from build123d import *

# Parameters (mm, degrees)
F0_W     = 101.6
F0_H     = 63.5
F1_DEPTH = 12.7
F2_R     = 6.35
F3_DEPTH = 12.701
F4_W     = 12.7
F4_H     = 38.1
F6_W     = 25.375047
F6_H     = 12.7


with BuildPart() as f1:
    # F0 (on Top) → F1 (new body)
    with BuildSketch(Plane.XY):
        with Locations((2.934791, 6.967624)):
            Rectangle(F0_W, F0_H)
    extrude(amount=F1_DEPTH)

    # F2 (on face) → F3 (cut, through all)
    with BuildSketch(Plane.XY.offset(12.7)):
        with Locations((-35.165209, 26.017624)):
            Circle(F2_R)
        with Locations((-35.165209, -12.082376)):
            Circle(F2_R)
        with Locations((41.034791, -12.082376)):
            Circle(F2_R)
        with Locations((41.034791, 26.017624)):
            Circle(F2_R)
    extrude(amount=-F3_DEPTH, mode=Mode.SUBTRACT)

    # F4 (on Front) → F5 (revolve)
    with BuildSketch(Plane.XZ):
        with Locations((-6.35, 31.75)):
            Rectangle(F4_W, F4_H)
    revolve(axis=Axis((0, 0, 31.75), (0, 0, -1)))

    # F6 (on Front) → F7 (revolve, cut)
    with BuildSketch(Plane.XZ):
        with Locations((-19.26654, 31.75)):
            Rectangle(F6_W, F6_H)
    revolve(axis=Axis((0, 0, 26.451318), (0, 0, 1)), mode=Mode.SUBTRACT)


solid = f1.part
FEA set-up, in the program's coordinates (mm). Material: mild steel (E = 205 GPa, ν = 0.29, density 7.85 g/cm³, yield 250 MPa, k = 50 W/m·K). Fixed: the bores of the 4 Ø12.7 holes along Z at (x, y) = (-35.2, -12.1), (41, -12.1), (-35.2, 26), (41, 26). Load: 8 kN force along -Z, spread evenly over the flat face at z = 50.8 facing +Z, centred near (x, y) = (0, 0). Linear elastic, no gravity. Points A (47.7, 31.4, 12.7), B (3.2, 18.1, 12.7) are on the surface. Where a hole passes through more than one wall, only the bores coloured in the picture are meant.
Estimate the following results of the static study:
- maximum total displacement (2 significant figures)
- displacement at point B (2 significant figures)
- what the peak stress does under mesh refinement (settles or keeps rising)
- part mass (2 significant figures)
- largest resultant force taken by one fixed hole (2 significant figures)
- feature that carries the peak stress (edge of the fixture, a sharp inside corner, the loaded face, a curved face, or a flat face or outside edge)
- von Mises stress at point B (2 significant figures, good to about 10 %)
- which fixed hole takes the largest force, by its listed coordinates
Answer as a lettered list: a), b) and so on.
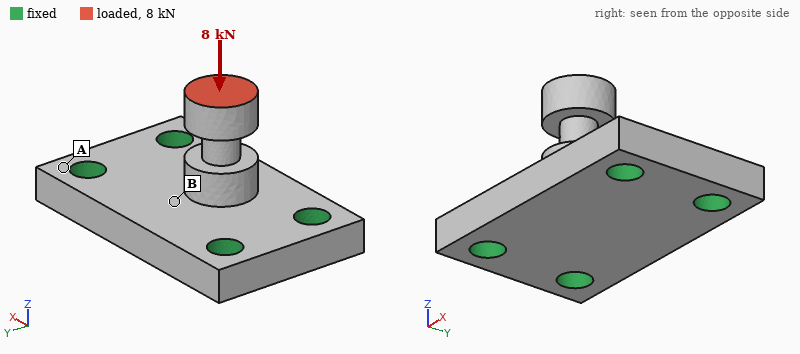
a) 16 µm
b) 5.9 µm
c) keeps rising
d) 710 g
e) 3.0 kN
f) edge of the fixture
g) 17 MPa
h) (-35.2, -12.1)
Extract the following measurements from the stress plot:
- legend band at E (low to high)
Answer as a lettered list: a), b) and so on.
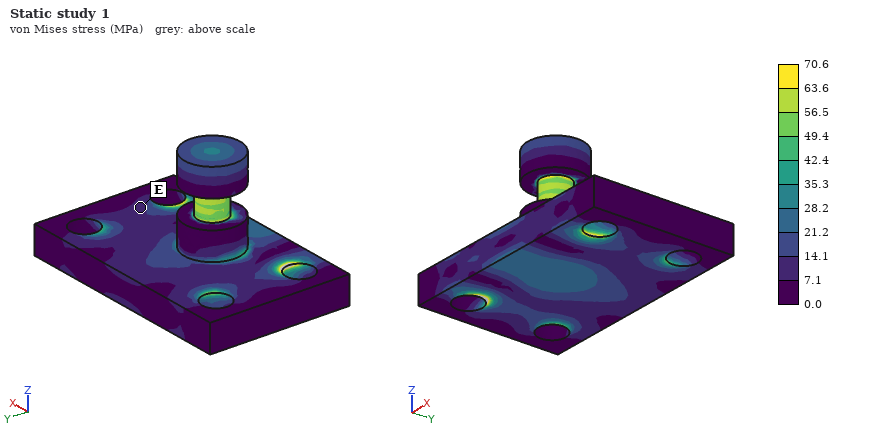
a) 7.1 to 14.1 MPa
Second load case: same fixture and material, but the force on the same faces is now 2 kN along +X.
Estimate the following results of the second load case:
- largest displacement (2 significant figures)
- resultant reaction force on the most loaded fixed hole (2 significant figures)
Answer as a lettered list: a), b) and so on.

a) 73 µm
b) 1.4 kN
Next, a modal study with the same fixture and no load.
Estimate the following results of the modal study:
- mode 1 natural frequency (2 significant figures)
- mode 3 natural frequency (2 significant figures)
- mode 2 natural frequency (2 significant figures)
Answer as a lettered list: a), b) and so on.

a) 4600 Hz
b) 9100 Hz
c) 4800 Hz
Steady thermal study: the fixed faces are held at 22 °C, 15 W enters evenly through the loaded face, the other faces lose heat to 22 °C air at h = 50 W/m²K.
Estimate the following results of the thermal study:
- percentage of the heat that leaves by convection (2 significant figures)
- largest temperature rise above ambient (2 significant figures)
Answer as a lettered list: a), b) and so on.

a) 35 %
b) 46 K
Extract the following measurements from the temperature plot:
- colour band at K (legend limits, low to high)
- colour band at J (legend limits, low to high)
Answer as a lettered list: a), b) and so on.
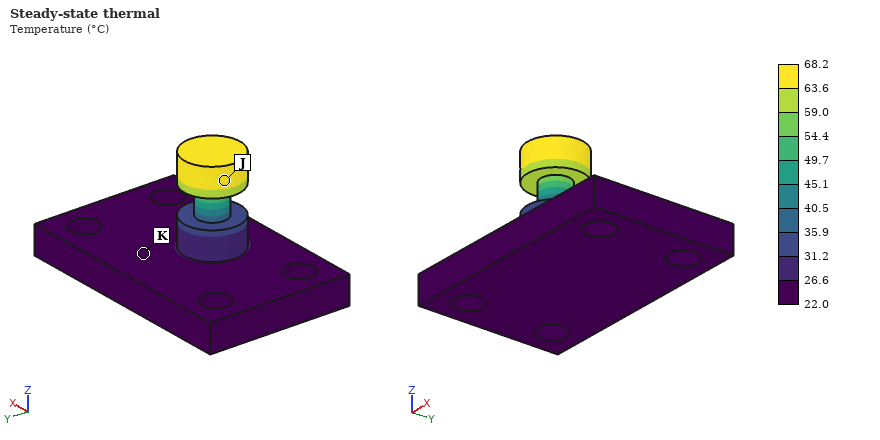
a) 22.0 to 26.6 °C
b) 63.6 to 68.2 °C
